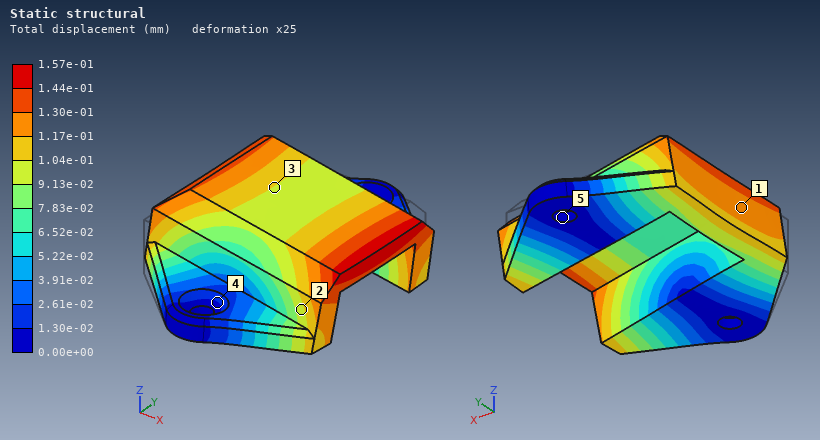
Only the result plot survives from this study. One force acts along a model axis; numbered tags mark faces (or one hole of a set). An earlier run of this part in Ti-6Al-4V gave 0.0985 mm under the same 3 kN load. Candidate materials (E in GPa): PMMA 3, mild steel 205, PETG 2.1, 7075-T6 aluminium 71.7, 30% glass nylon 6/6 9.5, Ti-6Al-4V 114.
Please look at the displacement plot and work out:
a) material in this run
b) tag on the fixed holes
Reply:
7075-T6 aluminium
5
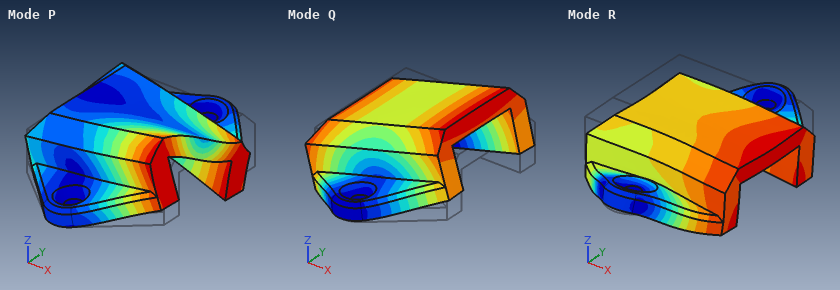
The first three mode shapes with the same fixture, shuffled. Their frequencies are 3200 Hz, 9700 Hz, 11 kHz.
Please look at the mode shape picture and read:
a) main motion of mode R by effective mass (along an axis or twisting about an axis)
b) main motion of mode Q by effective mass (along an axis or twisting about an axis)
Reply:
along Z
along X
